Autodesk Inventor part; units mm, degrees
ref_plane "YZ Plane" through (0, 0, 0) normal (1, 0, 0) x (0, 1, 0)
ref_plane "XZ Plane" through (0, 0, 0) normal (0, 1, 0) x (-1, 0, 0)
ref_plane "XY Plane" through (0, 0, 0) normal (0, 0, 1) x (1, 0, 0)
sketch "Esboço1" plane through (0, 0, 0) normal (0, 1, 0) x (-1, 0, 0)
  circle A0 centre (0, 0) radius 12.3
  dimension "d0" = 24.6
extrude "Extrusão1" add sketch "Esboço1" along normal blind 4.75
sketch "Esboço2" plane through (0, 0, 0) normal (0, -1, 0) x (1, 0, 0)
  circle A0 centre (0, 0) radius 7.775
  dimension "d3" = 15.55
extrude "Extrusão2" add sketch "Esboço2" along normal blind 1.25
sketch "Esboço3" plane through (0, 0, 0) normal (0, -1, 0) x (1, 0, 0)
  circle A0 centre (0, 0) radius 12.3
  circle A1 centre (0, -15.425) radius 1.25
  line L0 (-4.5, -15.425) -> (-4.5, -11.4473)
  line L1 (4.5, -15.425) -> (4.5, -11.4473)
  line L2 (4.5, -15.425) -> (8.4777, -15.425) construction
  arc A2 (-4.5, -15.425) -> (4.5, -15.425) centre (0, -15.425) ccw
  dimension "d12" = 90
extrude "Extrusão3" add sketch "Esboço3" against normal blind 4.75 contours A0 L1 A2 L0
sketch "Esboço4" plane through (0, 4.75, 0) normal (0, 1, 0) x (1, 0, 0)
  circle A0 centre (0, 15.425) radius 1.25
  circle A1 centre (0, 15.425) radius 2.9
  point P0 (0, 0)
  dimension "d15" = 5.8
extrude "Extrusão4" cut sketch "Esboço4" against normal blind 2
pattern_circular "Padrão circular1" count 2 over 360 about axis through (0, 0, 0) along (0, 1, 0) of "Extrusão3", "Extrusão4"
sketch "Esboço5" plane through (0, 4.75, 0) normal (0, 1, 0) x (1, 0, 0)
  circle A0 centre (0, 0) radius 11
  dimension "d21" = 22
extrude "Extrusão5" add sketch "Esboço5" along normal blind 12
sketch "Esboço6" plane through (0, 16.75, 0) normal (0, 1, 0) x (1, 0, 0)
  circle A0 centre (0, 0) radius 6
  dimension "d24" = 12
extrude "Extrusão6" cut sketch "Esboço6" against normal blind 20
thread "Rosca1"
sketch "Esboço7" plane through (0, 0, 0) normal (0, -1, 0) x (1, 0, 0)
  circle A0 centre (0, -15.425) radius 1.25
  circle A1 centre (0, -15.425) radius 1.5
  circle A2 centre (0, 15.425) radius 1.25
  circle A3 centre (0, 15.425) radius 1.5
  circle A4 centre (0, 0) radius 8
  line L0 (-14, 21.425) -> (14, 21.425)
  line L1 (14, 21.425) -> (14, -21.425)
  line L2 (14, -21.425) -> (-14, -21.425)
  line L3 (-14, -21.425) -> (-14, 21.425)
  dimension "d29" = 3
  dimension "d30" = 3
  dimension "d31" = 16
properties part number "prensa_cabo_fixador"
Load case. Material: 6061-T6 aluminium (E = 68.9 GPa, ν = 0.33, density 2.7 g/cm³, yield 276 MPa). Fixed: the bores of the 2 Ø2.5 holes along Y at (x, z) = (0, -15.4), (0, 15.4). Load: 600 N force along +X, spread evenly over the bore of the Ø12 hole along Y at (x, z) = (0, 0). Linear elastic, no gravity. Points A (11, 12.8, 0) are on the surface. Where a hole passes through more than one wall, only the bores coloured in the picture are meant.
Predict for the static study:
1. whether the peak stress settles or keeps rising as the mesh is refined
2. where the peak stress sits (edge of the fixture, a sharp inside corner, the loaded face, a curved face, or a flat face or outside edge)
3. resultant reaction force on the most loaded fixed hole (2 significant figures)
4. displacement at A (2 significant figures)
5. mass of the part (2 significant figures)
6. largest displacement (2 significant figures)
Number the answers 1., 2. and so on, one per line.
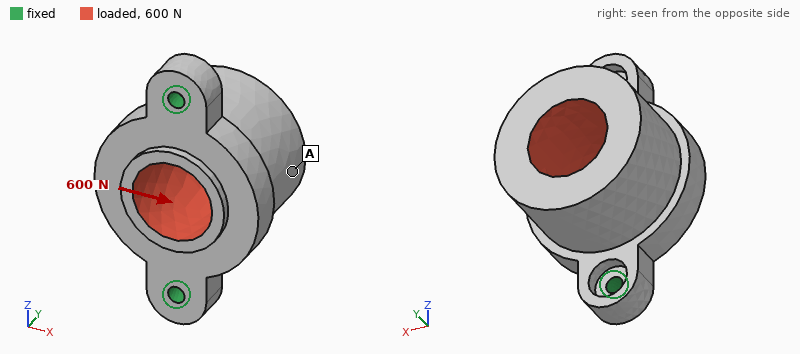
1. keeps rising
2. edge of the fixture
3. 300 N
4. 55 µm
5. 15 g
6. 65 µm
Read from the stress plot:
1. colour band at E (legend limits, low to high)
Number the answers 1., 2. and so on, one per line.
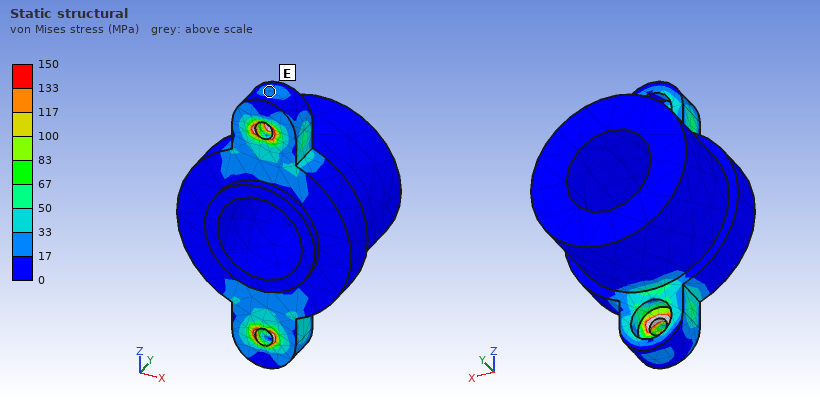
1. 17 to 33 MPa
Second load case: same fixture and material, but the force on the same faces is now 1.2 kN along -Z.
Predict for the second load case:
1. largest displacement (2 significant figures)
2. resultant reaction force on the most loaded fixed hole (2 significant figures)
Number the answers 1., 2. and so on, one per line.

1. 6.9 µm
2. 660 N
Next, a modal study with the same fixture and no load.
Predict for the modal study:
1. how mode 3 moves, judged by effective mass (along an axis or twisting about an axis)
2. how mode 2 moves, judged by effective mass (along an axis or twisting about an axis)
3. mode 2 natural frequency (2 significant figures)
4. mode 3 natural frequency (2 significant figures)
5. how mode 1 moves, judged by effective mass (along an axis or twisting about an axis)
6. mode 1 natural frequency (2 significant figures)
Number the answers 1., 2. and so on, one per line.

1. along Z
2. along Y
3. 14 kHz
4. 20 kHz
5. along X
6. 4400 Hz
